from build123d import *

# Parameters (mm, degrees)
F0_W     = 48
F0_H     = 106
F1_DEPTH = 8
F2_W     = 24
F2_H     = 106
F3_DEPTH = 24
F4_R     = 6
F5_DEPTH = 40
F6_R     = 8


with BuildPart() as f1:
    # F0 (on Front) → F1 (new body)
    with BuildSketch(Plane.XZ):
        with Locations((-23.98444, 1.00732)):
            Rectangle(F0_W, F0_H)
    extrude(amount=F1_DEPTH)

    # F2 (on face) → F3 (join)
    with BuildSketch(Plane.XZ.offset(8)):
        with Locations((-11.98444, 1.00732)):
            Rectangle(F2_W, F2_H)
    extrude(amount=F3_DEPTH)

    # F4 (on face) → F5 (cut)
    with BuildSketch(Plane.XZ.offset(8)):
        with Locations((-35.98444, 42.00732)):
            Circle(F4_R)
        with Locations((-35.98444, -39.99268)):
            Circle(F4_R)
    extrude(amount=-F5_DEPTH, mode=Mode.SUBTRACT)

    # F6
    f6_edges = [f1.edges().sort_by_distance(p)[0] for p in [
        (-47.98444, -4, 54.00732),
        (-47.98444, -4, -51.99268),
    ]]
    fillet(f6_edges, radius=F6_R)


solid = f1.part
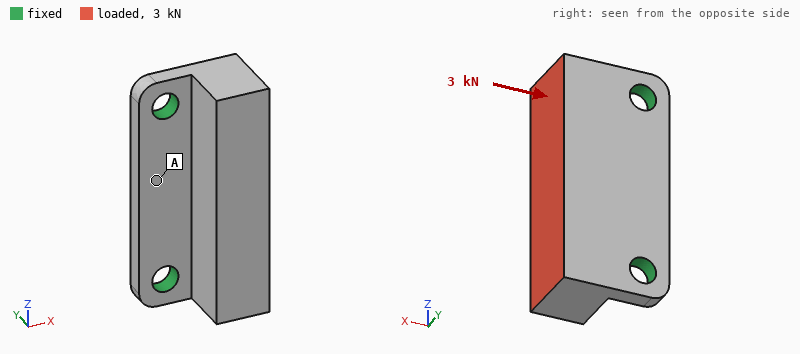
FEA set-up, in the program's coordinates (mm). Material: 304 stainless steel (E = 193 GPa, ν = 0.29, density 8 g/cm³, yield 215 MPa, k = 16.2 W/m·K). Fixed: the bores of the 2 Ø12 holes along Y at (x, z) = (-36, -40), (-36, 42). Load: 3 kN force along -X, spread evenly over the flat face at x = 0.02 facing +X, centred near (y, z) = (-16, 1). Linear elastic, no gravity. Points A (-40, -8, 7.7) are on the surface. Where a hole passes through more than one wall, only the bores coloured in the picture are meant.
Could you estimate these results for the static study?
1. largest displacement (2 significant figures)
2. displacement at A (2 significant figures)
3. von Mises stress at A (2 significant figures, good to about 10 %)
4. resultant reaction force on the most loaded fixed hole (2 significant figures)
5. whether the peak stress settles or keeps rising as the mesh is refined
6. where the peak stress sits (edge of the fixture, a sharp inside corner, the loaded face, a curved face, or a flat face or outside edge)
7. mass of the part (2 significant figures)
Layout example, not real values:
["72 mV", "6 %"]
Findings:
["28 µm", "4.8 µm", "7.5 MPa", "1.5 kN", "keeps rising", "edge of the fixture", "800 g"]
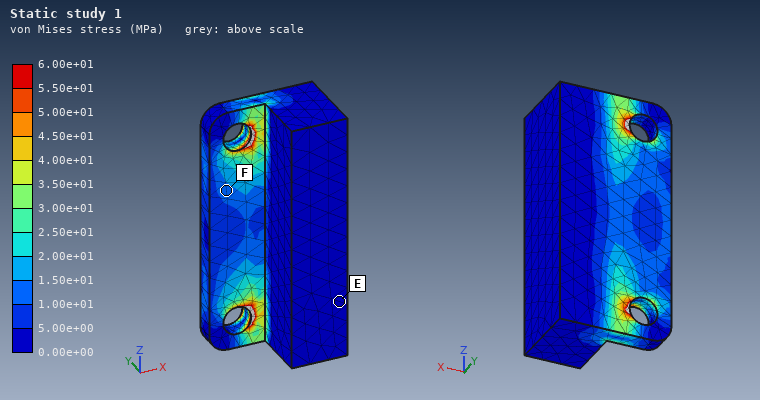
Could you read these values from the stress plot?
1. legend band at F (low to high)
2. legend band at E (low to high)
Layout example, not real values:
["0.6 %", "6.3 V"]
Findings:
["1.00e+01 to 1.50e+01 MPa", "0.00e+00 to 5.00e+00 MPa"]
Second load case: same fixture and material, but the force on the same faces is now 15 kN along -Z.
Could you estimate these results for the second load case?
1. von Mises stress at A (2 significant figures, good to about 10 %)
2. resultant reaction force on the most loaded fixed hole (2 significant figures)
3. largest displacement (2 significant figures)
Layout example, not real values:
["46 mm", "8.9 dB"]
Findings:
["12 MPa", "9.8 kN", "13 µm"]
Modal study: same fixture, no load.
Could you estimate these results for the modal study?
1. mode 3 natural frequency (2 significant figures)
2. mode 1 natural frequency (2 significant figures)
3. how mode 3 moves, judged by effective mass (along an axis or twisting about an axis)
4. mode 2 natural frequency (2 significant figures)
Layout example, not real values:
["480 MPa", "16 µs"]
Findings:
["7700 Hz", "1900 Hz", "along Y", "5900 Hz"]
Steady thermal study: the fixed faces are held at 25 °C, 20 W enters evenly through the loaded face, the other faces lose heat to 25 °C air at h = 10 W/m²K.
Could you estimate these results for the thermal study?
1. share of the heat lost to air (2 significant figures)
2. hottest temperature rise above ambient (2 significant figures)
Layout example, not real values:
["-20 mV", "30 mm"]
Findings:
["18 %", "38 K"]
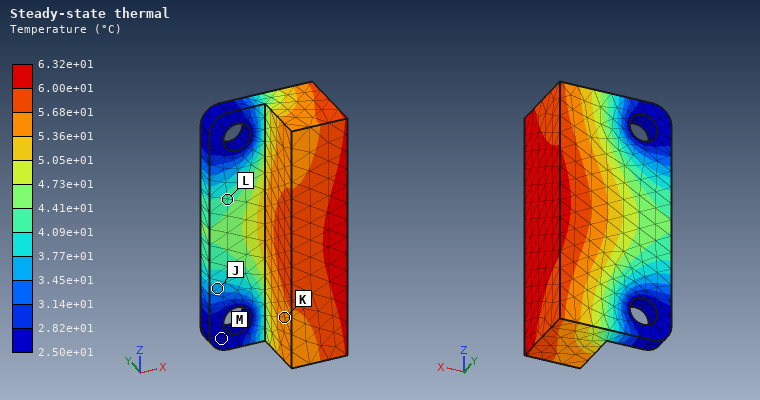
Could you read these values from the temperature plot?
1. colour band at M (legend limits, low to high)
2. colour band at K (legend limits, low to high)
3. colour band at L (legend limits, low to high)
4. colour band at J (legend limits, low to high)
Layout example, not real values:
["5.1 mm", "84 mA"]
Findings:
["2.50e+01 to 2.82e+01 °C", "5.36e+01 to 5.68e+01 °C", "4.09e+01 to 4.41e+01 °C", "3.45e+01 to 3.77e+01 °C"]
